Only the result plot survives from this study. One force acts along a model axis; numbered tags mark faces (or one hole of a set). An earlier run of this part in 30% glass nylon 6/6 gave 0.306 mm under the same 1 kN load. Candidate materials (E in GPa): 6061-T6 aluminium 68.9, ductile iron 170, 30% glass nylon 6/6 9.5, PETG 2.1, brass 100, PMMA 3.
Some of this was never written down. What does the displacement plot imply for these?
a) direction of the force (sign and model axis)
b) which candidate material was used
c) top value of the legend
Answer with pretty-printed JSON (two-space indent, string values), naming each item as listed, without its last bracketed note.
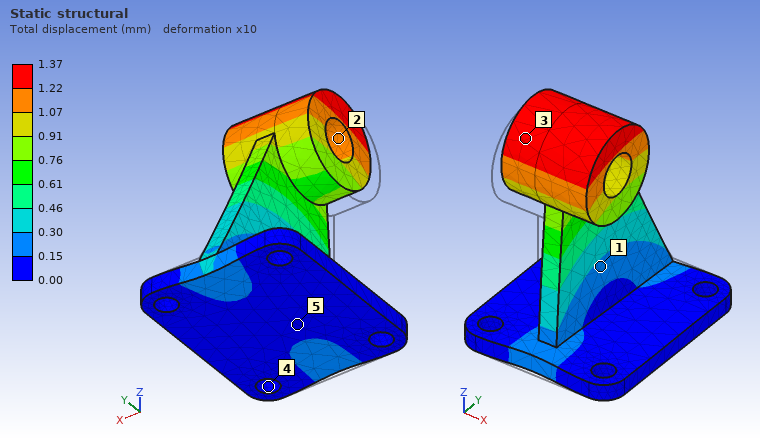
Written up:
{
  "direction of the force": "+Y",
  "which candidate material was used": "PETG",
  "top value of the legend": "1.37 mm"
}
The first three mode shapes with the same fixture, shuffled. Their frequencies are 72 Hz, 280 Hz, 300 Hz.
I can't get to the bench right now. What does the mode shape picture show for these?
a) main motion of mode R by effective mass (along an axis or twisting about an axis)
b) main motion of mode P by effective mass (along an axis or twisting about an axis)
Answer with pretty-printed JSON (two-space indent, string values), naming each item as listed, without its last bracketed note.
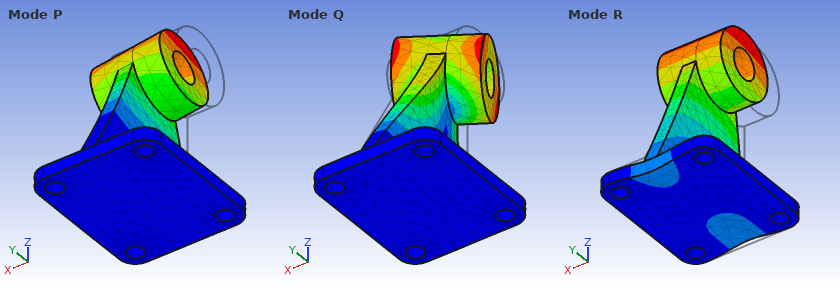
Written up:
{
  "main motion of mode R by effective mass": "along Y",
  "main motion of mode P by effective mass": "along X"
}
